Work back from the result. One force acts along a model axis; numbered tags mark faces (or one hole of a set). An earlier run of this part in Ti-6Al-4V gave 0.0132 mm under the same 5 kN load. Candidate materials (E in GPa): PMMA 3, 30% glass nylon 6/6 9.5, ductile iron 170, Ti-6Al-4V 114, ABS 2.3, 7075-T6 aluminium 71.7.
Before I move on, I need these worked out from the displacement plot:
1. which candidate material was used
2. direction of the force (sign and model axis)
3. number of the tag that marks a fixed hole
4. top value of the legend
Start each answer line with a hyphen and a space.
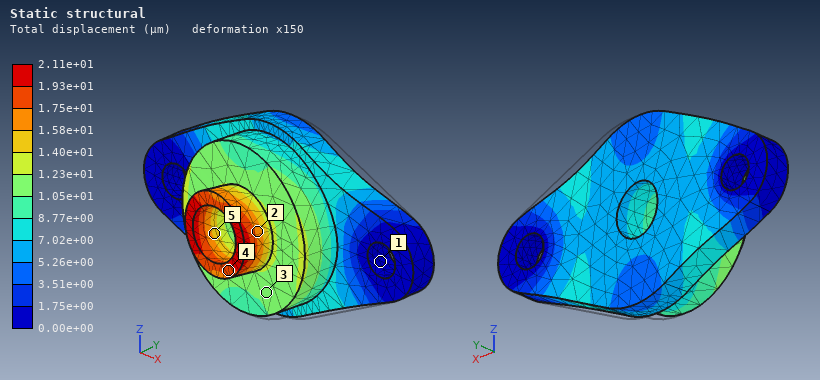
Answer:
- 7075-T6 aluminium
- -X
- 1
- 2.11e+01 µm
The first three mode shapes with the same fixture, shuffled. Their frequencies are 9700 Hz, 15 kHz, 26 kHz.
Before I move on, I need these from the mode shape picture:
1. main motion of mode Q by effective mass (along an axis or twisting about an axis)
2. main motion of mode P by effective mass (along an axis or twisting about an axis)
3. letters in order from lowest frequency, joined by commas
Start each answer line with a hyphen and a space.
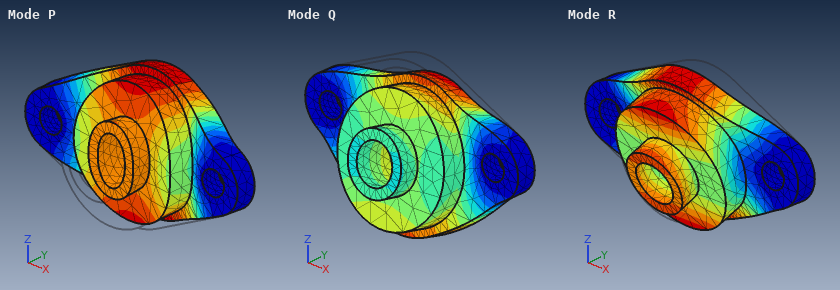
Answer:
- along Z
- along Y
- R, P, Q
